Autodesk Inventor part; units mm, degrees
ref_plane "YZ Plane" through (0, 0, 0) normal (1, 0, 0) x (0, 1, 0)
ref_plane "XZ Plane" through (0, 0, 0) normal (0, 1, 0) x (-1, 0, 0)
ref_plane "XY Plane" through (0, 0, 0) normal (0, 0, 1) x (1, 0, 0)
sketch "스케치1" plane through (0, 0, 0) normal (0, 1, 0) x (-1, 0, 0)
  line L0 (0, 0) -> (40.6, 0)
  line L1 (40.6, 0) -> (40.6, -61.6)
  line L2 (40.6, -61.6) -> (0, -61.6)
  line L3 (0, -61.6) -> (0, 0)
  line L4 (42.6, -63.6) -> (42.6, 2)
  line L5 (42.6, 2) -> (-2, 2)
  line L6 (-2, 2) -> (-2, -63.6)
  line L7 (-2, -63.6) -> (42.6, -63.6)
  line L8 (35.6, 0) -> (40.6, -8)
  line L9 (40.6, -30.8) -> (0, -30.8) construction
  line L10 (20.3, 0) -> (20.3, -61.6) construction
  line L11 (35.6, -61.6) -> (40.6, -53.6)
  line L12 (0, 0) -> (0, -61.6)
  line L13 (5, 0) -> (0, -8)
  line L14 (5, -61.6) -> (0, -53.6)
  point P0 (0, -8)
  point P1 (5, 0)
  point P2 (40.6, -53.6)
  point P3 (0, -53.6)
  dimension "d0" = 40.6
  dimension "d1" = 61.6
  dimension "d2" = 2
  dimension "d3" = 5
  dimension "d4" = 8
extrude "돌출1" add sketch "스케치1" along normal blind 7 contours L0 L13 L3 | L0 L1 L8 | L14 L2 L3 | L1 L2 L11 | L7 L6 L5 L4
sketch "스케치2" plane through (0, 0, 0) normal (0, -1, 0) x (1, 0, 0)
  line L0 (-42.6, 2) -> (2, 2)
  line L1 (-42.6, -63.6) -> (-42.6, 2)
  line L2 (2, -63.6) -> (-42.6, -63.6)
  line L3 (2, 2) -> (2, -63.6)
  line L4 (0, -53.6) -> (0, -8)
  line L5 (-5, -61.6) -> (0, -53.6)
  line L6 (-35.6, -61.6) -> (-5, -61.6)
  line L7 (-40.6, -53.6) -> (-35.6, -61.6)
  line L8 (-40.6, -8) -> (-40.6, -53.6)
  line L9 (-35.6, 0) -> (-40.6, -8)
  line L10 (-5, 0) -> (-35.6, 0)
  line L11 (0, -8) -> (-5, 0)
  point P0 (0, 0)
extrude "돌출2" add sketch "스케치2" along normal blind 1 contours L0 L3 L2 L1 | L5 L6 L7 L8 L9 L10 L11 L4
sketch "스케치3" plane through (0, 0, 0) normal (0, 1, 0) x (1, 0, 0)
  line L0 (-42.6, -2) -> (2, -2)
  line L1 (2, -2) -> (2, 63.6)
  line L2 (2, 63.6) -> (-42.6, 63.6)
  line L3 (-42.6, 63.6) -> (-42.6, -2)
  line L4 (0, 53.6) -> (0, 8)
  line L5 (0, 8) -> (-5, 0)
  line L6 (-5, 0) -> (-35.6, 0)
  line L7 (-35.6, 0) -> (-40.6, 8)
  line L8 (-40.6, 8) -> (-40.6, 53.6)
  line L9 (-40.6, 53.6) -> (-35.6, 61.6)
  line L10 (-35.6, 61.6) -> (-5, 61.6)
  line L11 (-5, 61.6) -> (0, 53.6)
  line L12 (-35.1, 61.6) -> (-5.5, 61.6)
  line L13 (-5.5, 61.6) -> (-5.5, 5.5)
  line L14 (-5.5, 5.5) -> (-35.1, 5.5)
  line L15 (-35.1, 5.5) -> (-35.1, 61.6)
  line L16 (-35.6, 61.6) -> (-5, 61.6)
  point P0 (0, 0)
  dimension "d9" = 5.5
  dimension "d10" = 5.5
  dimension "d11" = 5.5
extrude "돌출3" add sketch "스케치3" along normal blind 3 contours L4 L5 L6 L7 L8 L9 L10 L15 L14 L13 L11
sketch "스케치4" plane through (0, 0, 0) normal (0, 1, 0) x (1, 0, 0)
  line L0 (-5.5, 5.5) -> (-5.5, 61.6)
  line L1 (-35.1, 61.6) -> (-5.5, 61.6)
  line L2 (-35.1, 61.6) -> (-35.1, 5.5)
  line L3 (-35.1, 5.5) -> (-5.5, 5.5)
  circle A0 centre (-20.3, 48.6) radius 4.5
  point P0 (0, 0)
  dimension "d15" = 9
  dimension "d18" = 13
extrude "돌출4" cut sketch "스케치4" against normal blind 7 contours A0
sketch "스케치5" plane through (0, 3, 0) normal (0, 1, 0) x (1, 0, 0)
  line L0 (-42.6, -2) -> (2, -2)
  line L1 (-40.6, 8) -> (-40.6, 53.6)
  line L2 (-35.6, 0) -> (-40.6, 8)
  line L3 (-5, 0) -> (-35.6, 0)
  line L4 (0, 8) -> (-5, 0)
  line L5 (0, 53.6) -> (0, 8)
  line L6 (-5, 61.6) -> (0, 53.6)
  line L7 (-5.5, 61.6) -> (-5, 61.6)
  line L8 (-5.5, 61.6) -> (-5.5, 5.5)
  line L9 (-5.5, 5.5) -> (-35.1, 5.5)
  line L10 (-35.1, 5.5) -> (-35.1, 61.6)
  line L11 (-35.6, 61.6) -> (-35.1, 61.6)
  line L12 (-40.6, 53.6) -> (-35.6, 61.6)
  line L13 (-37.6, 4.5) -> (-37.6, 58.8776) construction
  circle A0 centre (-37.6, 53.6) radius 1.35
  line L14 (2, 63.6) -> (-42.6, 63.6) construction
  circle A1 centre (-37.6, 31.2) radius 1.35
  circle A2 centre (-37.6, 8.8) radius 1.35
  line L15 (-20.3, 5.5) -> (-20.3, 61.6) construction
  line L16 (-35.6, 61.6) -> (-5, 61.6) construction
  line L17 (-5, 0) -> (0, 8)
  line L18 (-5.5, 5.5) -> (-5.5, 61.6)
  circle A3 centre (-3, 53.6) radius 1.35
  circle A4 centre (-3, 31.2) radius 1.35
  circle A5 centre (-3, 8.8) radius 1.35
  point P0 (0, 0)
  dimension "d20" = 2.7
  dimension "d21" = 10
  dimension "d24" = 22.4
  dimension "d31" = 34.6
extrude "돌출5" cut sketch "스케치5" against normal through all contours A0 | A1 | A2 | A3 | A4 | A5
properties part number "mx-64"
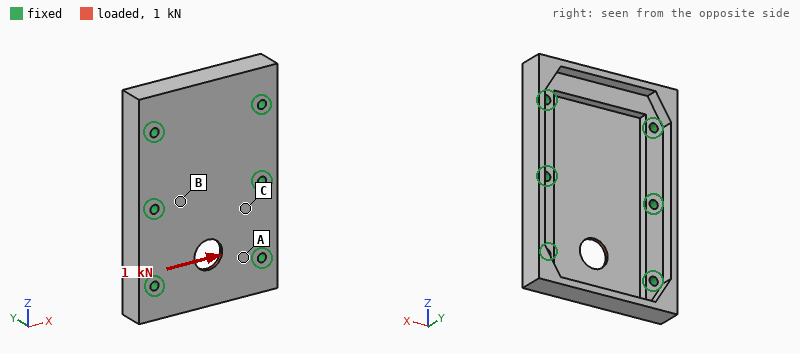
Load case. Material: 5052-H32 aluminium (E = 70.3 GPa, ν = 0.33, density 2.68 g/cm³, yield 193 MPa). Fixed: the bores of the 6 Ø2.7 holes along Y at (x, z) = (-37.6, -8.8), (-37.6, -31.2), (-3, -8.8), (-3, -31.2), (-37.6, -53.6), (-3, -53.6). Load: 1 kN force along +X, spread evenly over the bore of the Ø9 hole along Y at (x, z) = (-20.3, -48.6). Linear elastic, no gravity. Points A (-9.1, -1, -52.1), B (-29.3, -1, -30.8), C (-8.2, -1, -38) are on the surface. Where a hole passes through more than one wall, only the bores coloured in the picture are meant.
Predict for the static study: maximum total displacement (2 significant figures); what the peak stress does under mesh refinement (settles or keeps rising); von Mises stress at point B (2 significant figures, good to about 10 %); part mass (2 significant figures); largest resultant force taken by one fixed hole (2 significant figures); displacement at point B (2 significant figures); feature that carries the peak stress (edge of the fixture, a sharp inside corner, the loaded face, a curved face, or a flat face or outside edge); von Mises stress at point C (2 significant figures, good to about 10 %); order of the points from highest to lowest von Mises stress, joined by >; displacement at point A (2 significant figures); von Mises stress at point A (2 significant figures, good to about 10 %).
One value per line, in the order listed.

6.6 µm
keeps rising
5.7 MPa
23 g
350 N
1.0 µm
a sharp inside corner
13 MPa
A > C > B
2.9 µm
29 MPa
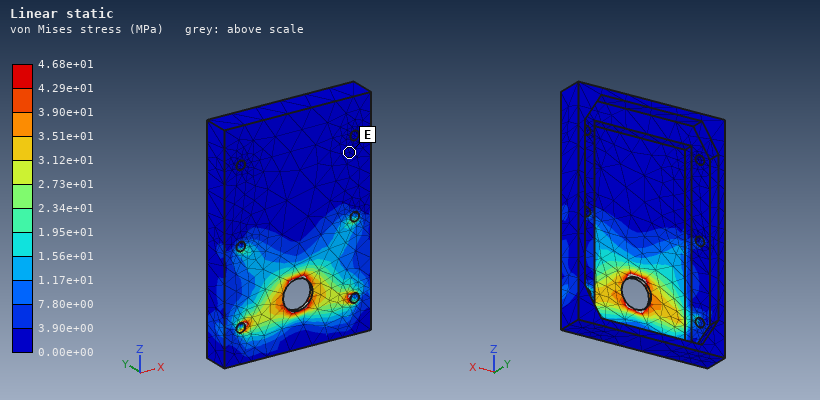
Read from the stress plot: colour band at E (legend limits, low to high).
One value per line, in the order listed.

0.00e+00 to 3.90e+00 MPa
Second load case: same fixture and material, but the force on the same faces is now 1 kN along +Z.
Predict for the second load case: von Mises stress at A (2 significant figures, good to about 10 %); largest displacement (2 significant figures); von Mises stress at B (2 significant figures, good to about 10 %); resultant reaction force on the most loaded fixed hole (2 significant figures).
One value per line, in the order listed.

21 MPa
12 µm
13 MPa
260 N
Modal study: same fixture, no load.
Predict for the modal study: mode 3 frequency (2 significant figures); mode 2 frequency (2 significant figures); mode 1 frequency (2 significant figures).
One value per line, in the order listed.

12 kHz
8800 Hz
6500 Hz
